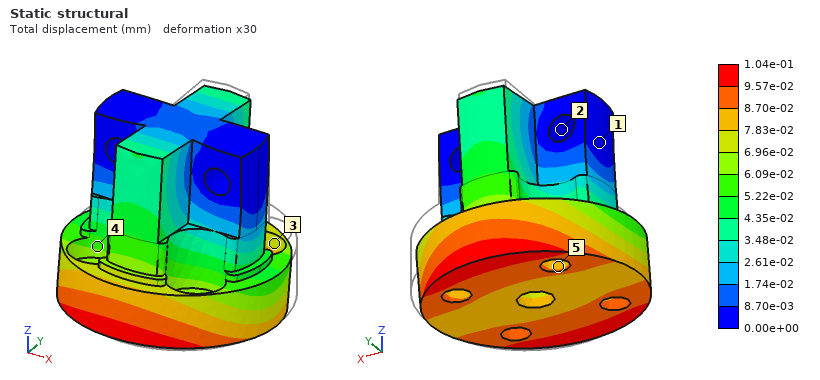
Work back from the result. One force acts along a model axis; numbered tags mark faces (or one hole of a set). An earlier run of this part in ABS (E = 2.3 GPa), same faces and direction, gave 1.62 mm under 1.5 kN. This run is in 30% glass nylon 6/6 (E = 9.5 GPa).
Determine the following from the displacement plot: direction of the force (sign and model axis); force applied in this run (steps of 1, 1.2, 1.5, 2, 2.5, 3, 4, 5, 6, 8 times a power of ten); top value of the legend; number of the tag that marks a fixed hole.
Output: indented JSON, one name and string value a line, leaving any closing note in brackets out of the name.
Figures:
{
  "direction of the force": "-Y",
  "force applied in this run": "400 N",
  "top value of the legend": "1.04e-01 mm",
  "number of the tag that marks a fixed hole": "2"
}
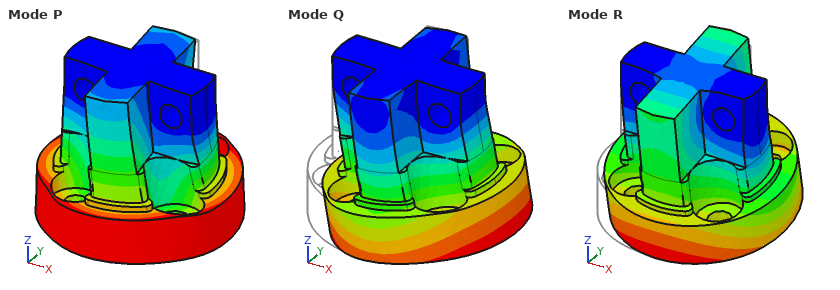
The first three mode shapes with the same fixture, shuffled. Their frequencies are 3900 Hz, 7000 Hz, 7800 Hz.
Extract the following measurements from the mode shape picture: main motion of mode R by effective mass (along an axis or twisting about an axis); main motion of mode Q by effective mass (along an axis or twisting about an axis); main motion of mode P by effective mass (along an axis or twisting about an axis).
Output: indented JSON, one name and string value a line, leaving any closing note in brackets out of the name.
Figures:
{
  "main motion of mode R by effective mass": "along Y",
  "main motion of mode Q by effective mass": "along X",
  "main motion of mode P by effective mass": "twisting about Z"
}
